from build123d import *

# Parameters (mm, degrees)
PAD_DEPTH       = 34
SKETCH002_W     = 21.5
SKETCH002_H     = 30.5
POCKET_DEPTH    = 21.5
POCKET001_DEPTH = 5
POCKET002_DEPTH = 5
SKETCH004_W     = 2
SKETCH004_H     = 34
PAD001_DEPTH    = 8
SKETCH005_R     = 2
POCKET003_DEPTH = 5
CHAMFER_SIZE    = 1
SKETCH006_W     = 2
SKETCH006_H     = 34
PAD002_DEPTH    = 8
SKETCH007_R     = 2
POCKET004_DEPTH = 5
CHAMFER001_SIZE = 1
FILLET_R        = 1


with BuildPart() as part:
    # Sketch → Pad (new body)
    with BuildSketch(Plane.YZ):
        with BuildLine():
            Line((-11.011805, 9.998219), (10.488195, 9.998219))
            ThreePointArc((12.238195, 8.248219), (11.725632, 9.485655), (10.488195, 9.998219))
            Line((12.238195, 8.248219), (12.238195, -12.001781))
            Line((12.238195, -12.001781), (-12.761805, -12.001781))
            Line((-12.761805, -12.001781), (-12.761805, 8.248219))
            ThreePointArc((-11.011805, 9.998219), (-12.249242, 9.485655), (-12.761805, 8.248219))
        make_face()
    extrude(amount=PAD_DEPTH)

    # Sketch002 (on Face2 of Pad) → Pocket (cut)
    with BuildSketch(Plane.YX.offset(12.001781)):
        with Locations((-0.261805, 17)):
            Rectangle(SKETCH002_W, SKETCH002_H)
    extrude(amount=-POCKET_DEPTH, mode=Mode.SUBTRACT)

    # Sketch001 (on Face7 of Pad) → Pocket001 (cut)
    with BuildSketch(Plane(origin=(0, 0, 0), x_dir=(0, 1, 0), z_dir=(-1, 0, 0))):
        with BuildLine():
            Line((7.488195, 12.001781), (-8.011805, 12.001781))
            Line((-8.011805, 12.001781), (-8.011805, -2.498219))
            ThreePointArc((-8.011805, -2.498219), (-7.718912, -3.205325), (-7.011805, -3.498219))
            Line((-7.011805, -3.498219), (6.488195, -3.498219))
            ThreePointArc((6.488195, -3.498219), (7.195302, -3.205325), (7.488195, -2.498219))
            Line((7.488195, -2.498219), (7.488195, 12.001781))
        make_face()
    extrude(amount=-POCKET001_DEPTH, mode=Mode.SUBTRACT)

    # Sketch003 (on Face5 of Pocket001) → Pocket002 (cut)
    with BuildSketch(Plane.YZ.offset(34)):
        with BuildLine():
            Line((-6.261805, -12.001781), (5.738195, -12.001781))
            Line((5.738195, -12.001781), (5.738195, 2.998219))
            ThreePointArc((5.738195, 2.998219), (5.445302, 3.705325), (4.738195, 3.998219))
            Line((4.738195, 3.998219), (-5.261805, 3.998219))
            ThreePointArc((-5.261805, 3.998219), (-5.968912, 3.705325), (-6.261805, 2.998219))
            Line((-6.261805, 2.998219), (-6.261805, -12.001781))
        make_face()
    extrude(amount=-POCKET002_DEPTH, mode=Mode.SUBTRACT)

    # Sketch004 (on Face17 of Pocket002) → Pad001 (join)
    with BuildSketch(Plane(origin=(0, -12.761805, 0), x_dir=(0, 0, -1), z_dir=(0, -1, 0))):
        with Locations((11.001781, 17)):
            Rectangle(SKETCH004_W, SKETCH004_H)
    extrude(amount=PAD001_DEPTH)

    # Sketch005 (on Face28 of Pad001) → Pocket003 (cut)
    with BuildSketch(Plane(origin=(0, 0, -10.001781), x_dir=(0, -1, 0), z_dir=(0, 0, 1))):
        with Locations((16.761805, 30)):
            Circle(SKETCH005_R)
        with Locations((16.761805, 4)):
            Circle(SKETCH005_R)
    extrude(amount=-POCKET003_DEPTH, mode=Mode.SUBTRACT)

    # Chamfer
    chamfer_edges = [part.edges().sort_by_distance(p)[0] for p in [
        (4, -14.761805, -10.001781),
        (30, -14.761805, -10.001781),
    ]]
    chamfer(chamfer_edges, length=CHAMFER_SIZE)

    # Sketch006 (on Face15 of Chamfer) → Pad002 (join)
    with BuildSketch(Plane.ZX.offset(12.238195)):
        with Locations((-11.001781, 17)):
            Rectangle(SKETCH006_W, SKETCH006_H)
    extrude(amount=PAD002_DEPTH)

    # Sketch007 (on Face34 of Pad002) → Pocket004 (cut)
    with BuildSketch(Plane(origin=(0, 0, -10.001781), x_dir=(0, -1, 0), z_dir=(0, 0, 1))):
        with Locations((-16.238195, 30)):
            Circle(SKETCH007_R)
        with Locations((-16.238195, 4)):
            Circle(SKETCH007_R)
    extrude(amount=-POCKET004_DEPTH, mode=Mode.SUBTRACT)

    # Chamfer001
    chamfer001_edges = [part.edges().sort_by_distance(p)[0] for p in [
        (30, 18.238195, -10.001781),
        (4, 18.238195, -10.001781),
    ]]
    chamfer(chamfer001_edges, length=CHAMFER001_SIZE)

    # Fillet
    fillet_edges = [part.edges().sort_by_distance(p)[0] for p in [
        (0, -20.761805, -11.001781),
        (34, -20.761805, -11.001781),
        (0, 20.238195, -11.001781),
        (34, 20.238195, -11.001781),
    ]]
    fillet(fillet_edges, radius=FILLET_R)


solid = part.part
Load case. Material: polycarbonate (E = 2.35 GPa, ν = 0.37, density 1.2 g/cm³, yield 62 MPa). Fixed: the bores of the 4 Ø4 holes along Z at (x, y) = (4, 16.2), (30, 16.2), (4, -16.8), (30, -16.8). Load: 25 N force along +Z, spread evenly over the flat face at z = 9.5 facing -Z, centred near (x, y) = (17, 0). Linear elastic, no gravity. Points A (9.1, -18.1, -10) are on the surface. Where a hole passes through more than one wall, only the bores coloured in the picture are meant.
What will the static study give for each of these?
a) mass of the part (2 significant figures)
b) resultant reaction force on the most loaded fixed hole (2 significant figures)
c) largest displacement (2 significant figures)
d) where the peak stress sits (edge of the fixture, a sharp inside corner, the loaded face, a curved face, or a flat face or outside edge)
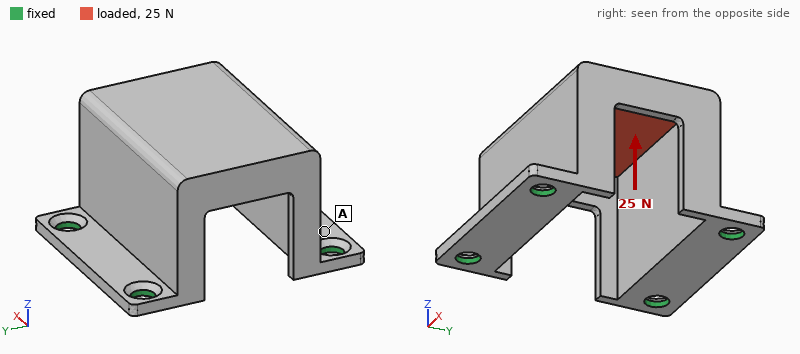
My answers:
5.7 g
6.7 N
0.67 mm
a curved face
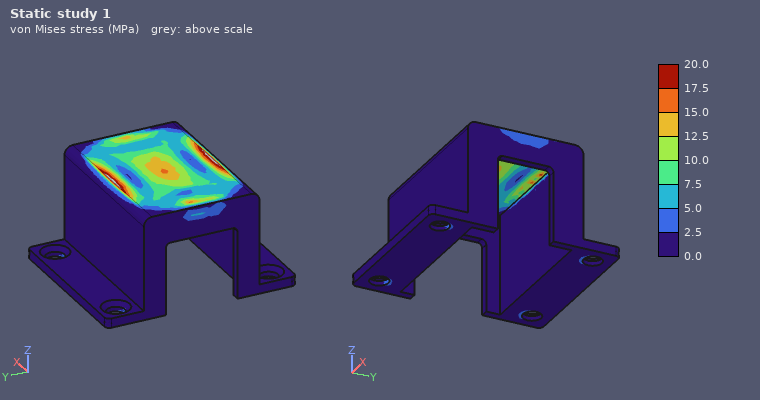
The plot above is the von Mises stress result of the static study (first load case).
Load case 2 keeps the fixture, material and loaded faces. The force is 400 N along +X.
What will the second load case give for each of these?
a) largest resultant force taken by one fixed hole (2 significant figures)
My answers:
190 N
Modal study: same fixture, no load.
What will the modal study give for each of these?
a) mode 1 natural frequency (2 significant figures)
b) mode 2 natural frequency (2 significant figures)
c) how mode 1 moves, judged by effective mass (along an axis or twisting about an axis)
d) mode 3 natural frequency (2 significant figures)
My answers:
1800 Hz
2000 Hz
along Y
2700 Hz
